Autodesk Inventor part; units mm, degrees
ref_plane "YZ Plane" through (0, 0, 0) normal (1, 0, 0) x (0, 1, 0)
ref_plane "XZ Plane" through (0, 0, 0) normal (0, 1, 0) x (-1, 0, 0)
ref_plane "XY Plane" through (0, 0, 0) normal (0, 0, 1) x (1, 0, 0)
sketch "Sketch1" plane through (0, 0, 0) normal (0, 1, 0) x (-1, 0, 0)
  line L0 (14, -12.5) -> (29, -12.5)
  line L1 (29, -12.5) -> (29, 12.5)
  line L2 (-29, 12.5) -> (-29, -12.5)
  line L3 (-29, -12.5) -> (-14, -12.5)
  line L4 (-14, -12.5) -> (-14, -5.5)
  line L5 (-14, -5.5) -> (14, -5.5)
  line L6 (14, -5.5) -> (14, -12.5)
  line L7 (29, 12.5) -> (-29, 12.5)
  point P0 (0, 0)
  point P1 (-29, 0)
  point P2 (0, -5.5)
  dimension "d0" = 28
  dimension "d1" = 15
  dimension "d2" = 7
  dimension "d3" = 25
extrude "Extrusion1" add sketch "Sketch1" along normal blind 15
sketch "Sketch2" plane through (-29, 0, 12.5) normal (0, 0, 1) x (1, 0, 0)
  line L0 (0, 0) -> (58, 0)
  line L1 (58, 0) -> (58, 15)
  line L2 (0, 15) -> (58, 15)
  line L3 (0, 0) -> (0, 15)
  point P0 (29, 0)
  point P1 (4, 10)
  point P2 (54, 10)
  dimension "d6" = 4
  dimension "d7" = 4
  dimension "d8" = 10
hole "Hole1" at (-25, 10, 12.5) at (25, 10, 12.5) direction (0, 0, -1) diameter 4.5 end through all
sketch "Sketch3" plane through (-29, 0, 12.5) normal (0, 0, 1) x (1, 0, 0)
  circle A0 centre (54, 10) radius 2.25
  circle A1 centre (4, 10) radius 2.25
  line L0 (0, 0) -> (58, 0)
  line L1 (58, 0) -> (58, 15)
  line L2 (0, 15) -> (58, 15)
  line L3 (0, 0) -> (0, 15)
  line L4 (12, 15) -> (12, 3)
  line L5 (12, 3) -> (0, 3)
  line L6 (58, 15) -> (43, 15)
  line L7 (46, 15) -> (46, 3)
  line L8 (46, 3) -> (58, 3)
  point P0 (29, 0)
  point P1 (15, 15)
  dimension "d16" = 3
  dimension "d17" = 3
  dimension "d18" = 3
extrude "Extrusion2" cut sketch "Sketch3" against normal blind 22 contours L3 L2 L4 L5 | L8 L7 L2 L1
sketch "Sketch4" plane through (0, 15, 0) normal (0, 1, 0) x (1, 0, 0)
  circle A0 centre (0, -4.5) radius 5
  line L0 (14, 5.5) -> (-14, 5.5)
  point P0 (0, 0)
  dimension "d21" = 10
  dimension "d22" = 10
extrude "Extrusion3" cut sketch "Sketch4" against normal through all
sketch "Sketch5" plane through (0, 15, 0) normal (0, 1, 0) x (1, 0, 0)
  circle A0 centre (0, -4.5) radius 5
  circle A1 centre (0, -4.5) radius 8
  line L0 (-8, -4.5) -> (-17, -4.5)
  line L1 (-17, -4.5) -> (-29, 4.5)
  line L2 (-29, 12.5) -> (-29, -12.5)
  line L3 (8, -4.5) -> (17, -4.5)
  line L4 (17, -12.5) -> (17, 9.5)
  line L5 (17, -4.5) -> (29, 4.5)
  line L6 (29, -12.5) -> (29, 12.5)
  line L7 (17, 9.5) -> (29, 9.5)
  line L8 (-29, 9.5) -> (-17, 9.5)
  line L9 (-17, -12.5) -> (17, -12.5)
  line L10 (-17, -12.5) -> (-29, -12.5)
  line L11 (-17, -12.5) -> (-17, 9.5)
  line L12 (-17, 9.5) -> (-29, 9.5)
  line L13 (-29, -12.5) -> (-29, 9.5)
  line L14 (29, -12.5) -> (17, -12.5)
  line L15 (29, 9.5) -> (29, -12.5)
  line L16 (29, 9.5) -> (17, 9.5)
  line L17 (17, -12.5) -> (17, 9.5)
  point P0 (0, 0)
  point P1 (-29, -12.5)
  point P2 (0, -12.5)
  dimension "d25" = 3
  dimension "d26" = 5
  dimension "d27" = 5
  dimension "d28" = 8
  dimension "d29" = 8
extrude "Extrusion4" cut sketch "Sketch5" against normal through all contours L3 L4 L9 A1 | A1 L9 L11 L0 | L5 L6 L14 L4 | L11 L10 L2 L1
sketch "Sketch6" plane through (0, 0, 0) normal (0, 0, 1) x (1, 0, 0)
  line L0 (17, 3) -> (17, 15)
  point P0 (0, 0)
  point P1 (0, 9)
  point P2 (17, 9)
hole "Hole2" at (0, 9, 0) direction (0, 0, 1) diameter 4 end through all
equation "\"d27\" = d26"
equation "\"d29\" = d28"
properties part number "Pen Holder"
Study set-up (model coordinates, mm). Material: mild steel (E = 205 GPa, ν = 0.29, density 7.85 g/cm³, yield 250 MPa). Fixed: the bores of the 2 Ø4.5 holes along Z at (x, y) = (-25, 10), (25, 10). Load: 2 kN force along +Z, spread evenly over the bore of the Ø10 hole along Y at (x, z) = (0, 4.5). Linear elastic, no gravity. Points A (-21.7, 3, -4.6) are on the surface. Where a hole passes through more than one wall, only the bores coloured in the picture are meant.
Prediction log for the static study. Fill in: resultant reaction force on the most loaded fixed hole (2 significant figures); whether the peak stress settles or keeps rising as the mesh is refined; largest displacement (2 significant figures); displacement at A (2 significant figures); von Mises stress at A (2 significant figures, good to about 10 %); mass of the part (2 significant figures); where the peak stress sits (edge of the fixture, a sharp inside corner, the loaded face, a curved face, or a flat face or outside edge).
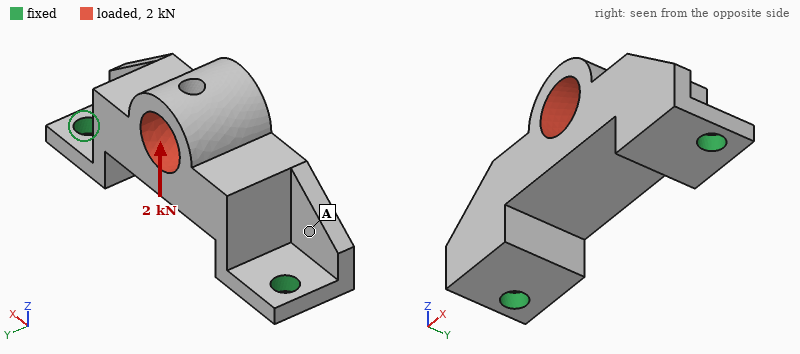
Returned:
1.4 kN
keeps rising
19 µm
9.3 µm
33 MPa
60 g
edge of the fixture
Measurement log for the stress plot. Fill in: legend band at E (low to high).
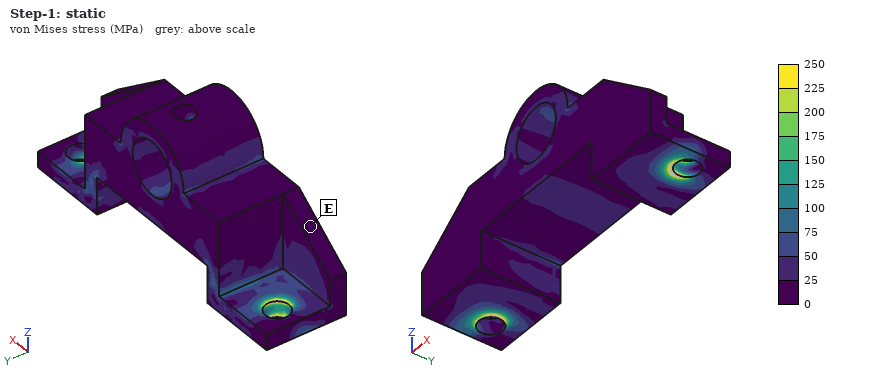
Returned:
0 to 25 MPa
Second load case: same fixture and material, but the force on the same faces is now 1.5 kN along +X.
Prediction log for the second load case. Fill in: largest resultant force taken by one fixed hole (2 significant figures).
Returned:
910 N
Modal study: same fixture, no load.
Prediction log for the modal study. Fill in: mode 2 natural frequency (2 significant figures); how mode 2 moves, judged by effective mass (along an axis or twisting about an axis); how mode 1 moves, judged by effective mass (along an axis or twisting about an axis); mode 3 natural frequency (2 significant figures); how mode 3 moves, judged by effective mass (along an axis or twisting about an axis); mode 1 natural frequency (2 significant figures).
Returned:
9400 Hz
along Z
along Y
11 kHz
along X
3400 Hz
